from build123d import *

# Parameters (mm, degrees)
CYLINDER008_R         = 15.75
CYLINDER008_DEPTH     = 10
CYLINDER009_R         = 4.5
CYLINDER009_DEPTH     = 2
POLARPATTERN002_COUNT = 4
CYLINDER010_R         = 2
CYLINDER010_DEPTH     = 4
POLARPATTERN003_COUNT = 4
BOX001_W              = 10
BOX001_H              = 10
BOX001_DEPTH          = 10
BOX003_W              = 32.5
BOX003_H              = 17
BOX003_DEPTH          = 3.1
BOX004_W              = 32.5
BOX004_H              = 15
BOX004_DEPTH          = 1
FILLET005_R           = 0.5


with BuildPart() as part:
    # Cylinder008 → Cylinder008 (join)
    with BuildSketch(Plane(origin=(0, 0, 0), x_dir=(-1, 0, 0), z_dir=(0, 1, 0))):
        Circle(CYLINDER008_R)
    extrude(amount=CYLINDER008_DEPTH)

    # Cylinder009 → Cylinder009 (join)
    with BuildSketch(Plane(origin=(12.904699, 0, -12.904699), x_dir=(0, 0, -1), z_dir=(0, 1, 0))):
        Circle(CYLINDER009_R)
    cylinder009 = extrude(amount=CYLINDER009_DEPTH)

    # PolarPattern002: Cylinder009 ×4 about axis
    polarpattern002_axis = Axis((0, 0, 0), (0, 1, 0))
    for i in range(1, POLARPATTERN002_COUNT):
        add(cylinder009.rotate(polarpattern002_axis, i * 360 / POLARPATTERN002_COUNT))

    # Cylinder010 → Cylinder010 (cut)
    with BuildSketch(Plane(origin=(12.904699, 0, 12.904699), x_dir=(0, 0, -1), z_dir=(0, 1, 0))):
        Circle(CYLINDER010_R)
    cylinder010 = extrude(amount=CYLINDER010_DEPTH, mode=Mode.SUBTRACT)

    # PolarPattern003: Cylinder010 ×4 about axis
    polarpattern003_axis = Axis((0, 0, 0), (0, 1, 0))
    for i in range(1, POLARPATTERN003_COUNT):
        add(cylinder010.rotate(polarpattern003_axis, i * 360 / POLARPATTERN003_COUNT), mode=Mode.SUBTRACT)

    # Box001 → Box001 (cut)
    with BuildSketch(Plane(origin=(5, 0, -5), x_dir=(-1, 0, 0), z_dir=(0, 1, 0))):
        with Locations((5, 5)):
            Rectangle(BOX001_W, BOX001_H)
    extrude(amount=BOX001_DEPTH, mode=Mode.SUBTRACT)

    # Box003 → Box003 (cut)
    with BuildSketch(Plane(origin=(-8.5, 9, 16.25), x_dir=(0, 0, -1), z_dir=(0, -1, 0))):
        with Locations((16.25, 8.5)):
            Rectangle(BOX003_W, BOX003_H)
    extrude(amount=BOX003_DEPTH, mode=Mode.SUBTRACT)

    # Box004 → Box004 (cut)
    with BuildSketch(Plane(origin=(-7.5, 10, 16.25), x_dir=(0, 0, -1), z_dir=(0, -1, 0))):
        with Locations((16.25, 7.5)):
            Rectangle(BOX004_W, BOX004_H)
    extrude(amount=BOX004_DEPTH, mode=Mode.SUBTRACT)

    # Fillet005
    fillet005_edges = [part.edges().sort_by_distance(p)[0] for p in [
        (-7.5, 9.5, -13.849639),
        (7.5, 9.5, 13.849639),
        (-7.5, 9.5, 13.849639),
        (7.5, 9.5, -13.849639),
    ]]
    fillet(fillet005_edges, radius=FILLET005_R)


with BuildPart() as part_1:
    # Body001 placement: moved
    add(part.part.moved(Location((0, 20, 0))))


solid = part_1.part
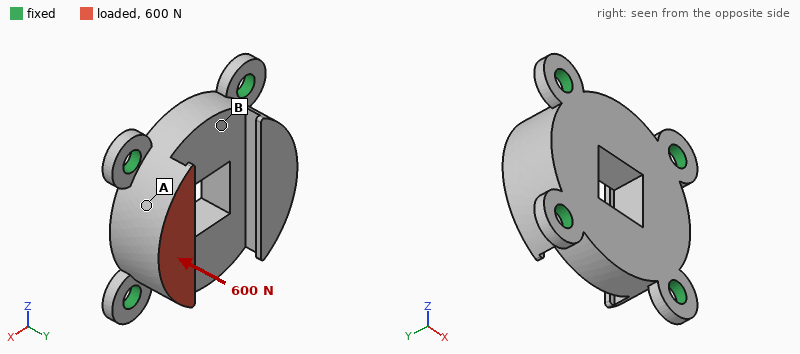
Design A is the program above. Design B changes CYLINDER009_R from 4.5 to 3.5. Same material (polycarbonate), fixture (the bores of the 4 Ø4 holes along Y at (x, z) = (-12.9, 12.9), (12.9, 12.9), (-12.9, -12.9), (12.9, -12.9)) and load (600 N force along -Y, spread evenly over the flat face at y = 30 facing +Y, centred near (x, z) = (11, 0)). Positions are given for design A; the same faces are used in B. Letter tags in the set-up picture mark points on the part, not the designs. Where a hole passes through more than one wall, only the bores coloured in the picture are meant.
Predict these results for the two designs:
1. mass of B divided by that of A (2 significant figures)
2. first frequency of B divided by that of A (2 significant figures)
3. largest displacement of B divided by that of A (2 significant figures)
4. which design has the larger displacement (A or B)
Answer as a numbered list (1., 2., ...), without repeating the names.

1. 0.97
2. 0.96
3. 1.1
4. B
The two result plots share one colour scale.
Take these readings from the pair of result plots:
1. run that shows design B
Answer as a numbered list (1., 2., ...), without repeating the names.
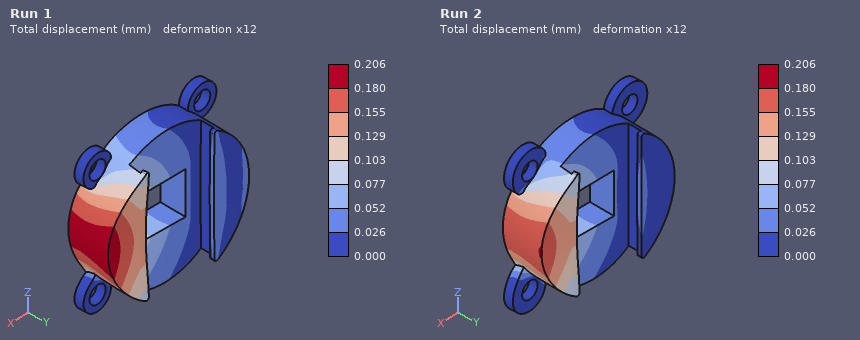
1. Run 1
